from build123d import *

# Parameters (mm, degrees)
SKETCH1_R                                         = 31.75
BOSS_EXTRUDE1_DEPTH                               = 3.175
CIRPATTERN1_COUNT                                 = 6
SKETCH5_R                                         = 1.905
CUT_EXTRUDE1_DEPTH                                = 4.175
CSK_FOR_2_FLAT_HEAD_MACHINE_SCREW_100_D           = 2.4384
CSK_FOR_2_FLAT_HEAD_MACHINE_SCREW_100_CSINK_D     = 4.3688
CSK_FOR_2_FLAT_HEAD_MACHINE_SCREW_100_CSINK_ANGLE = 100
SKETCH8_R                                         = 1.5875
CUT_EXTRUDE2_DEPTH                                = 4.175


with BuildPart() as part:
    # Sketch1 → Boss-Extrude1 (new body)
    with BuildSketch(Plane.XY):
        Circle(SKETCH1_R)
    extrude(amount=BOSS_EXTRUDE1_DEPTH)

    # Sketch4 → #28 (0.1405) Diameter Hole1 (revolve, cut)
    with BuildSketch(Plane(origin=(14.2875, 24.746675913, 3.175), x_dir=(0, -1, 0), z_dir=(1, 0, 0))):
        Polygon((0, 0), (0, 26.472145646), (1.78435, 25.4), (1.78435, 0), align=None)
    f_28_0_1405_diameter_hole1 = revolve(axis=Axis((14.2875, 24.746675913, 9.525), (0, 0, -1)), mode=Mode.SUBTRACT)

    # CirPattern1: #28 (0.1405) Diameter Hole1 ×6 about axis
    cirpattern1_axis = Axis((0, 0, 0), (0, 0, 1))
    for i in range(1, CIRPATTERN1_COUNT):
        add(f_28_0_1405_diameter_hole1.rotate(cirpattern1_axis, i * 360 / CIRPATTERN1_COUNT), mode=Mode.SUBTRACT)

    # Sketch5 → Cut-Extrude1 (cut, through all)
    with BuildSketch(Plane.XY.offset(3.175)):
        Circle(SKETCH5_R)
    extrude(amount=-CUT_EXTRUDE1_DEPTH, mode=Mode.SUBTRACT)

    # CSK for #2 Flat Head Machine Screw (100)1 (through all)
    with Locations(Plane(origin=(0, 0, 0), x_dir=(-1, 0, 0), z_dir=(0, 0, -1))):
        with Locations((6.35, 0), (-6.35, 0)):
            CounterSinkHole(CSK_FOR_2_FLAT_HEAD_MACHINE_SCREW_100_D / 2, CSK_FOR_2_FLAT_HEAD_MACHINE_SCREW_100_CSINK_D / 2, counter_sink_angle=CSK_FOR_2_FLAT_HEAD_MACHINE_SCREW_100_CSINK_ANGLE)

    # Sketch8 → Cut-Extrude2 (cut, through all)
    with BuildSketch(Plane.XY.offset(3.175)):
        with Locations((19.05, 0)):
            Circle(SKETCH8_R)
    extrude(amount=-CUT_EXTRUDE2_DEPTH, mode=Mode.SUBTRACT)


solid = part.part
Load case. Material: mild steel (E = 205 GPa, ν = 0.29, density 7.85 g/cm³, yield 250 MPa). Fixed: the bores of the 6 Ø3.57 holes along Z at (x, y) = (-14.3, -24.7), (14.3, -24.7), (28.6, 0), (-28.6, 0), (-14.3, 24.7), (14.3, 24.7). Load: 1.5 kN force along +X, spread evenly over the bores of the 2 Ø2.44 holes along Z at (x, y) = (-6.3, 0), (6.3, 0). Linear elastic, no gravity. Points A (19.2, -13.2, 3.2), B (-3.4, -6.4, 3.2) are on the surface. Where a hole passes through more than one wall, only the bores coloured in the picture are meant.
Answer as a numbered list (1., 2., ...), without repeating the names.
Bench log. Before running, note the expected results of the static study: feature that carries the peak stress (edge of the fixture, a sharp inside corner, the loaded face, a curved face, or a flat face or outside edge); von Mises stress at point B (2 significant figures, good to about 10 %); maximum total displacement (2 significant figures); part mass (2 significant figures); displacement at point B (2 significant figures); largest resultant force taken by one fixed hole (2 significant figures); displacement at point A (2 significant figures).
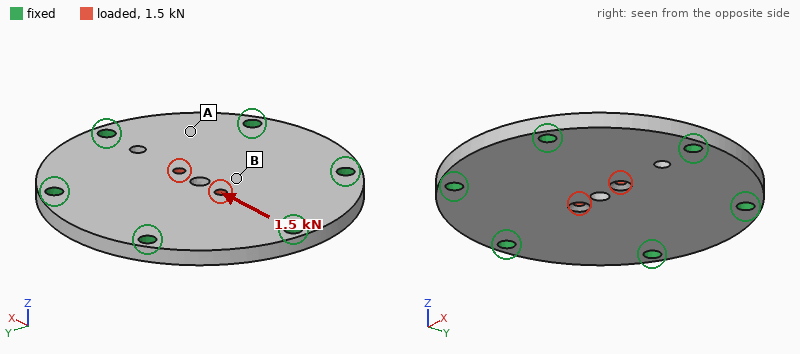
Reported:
1. the loaded face
2. 9.7 MPa
3. 1.9 µm
4. 77 g
5. 0.97 µm
6. 400 N
7. 0.50 µm
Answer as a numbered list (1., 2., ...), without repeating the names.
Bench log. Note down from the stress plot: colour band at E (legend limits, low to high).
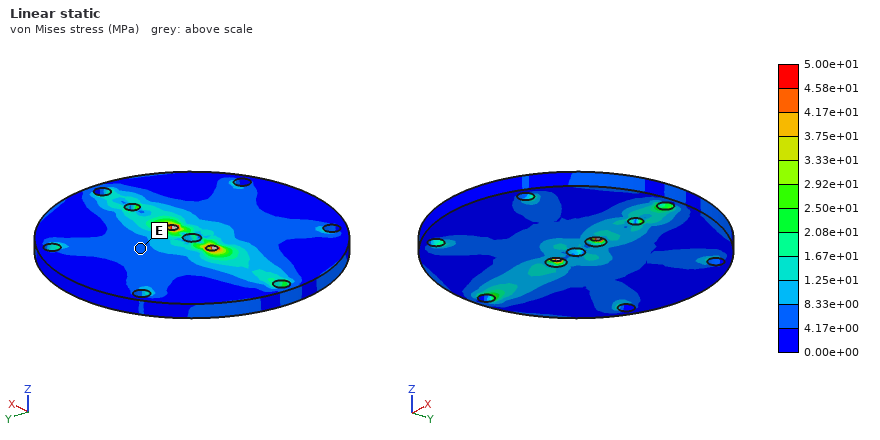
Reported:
1. 4.17e+00 to 8.33e+00 MPa
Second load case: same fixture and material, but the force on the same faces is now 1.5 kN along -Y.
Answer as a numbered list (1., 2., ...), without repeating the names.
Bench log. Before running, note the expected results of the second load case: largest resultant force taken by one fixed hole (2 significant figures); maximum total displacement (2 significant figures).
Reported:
1. 320 N
2. 1.6 µm
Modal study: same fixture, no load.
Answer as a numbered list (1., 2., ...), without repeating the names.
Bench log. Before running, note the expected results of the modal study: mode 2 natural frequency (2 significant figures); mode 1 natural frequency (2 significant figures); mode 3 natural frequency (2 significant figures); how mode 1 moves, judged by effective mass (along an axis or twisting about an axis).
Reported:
1. 16 kHz
2. 8100 Hz
3. 16 kHz
4. along Z
